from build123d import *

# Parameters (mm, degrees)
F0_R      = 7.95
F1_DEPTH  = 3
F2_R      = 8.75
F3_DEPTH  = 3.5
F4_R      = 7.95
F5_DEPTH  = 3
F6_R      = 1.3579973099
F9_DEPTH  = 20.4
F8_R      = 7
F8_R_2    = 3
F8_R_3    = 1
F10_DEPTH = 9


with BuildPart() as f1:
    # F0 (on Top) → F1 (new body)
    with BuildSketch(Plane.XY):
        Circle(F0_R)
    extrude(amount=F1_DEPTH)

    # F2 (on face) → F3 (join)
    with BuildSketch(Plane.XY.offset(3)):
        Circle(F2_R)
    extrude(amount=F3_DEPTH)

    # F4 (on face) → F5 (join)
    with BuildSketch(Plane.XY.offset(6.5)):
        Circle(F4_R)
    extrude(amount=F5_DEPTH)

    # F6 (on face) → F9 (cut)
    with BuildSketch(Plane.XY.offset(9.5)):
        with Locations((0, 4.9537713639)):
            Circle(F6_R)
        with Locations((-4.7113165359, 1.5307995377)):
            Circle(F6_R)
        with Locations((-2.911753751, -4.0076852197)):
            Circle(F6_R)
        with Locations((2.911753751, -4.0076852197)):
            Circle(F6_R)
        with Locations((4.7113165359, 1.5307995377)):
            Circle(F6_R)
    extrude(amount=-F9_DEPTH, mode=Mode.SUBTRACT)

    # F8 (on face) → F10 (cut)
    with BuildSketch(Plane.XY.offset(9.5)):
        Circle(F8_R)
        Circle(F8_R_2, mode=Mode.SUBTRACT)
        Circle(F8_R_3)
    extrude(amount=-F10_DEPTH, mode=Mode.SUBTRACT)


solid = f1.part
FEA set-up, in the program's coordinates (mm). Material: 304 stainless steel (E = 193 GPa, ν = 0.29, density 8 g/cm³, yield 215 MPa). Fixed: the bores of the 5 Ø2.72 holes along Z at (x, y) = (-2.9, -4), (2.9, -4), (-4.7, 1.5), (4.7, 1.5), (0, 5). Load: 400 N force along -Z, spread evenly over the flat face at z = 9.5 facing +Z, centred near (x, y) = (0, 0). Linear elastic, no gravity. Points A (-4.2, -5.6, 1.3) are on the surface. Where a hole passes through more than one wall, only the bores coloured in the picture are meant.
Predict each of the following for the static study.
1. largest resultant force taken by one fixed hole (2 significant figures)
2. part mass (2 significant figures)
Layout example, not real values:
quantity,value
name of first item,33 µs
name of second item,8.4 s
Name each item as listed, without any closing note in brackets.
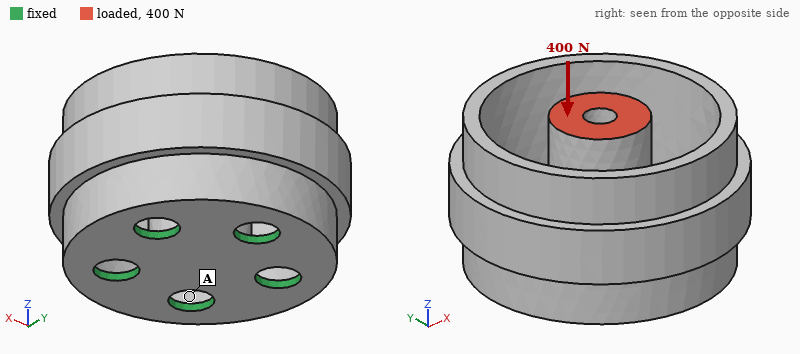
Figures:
quantity,value
largest resultant force taken by one fixed hole,92 N
part mass,6.9 g
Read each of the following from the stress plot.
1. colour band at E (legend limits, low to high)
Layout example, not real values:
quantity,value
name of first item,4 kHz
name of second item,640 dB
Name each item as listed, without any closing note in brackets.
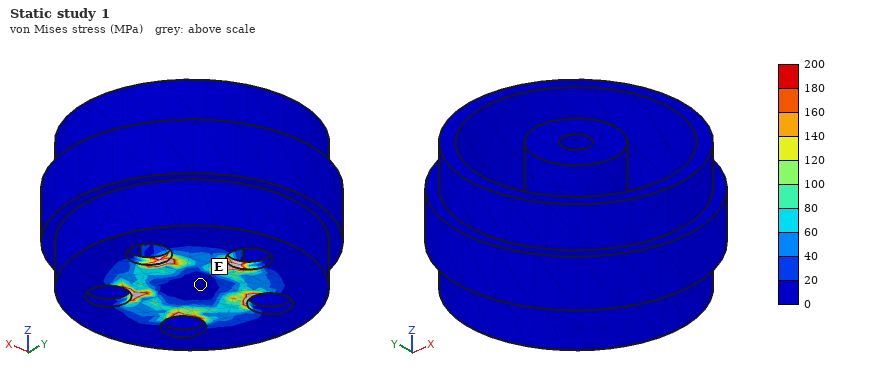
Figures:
quantity,value
colour band at E,0 to 20 MPa
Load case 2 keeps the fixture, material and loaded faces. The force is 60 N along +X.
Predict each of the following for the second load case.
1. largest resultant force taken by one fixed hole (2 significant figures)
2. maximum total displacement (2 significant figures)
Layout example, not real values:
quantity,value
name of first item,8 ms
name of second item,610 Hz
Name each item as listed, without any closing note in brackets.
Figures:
quantity,value
largest resultant force taken by one fixed hole,65 N
maximum total displacement,5.9 µm
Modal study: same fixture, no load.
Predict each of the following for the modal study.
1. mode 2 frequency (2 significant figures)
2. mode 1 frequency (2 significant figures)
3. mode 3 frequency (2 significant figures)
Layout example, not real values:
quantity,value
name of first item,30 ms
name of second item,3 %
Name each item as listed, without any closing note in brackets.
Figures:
quantity,value
mode 2 frequency,19 kHz
mode 1 frequency,19 kHz
mode 3 frequency,19 kHz
